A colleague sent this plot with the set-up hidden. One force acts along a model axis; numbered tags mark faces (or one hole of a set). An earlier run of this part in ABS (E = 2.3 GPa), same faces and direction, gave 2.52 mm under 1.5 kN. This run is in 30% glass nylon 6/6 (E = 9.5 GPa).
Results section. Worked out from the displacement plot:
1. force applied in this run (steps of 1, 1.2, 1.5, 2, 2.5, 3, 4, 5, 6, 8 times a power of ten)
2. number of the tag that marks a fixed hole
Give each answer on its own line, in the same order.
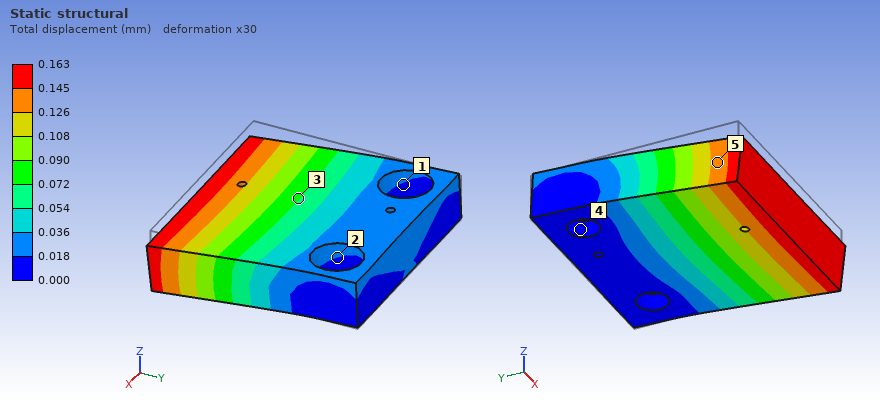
400 N
4
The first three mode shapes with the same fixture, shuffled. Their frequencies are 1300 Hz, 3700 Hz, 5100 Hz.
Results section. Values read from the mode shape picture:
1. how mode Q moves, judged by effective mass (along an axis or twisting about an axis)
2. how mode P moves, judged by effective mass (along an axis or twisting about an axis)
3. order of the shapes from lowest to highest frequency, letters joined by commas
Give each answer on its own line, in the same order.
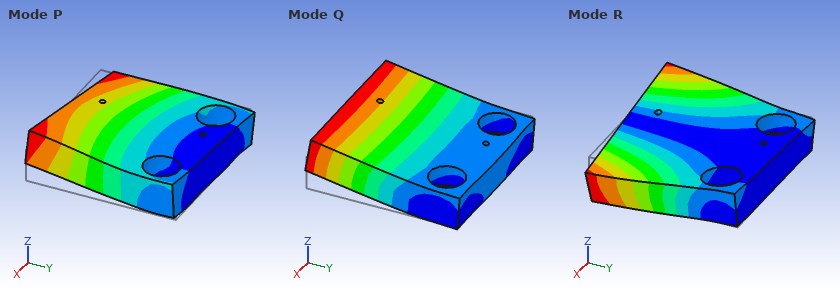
along Z
along X
Q, R, P
